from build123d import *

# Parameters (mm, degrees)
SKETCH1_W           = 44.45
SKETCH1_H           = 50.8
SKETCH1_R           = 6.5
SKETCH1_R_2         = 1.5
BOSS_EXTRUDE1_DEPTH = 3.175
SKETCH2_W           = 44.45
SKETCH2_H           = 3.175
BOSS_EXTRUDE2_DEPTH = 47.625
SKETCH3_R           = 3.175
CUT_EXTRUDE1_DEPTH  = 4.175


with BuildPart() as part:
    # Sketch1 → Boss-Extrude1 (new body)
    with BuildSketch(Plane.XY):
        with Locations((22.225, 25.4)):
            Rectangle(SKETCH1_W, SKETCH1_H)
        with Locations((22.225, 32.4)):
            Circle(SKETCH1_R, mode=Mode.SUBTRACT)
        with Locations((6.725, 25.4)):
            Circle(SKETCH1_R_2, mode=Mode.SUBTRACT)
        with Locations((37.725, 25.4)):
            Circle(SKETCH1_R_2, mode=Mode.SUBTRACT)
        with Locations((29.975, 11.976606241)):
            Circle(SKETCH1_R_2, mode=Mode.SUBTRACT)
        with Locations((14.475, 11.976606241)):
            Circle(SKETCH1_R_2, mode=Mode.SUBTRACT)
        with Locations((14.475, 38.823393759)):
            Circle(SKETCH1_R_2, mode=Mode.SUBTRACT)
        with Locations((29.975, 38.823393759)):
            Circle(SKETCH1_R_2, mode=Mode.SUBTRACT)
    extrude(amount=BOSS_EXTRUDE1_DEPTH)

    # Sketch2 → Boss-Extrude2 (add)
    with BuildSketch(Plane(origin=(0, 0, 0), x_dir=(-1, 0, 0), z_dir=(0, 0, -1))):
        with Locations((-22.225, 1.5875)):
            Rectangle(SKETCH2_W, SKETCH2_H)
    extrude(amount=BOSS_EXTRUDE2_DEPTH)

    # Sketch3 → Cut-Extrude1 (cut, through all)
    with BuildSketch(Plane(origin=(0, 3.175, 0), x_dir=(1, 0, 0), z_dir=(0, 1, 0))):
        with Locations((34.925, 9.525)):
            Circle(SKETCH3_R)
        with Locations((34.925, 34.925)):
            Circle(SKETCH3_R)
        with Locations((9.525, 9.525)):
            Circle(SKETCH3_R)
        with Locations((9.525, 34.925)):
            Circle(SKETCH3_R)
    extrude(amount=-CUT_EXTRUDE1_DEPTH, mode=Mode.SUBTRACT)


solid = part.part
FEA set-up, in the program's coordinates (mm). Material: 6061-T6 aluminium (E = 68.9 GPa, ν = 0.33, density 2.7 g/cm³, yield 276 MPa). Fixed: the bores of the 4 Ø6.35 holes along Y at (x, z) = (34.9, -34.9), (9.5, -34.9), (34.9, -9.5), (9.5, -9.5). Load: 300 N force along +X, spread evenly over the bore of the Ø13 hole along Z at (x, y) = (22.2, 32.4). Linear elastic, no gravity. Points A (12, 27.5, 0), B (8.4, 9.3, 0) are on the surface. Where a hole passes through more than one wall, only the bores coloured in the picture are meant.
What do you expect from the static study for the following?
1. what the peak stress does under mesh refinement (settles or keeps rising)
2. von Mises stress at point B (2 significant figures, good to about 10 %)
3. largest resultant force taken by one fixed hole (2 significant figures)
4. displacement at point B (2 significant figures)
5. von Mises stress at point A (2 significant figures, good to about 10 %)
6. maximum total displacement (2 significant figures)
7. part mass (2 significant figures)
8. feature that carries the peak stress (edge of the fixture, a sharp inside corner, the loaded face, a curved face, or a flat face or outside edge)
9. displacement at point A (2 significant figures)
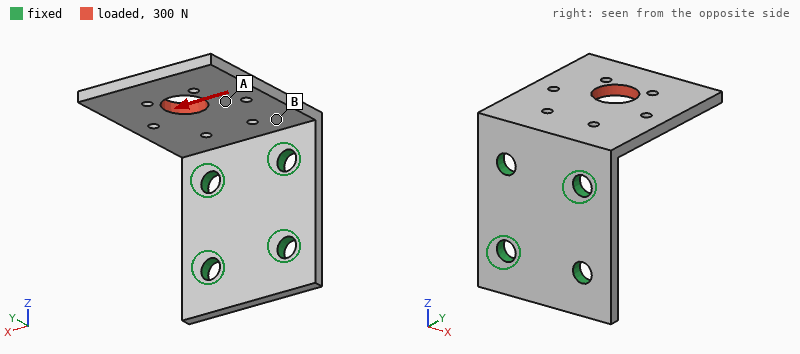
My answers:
keeps rising
19 MPa
370 N
22 µm
7.0 MPa
83 µm
35 g
edge of the fixture
42 µm
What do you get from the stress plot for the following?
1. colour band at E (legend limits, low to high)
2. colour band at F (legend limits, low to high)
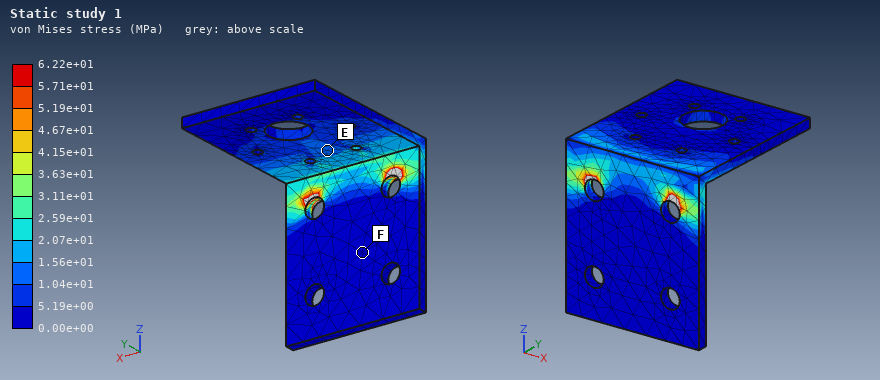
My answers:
1.04e+01 to 1.56e+01 MPa
0.00e+00 to 5.19e+00 MPa
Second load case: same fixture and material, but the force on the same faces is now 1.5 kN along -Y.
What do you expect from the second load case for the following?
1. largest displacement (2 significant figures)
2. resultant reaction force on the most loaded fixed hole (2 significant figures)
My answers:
0.41 mm
780 N
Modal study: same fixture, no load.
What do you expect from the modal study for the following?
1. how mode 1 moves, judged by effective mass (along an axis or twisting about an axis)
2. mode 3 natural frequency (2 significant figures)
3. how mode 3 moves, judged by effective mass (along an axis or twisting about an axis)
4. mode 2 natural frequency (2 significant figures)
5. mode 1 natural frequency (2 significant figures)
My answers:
along Z
3500 Hz
along X
2300 Hz
870 Hz
